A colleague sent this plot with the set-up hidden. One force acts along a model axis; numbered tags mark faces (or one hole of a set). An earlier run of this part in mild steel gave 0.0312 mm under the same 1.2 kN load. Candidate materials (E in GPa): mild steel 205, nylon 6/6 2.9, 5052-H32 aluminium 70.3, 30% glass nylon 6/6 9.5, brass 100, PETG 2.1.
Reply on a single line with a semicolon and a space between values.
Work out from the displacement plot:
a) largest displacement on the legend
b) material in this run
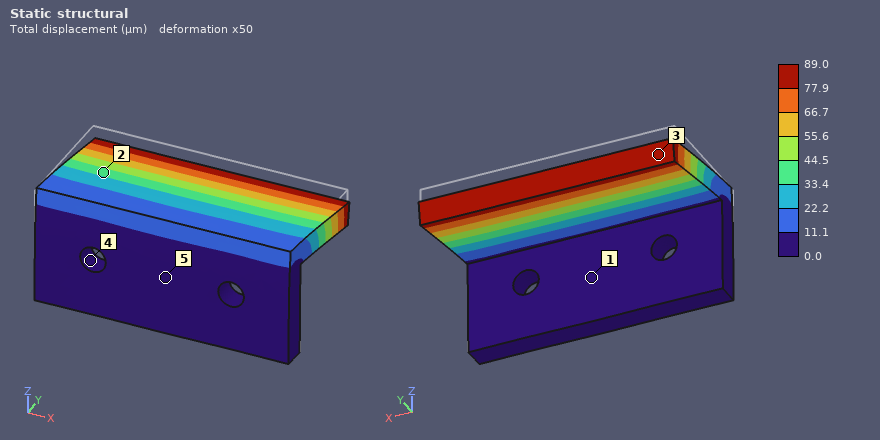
89.0 µm; 5052-H32 aluminium
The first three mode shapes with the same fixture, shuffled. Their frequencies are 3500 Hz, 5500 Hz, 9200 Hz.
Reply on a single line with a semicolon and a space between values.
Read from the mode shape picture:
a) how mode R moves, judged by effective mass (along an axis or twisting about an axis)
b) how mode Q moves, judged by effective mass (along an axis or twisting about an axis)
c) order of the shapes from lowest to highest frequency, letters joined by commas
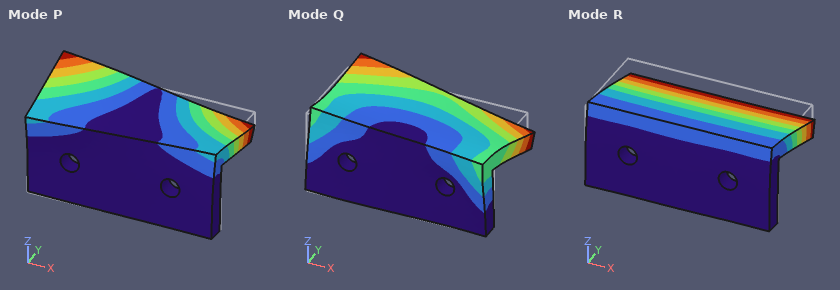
along Z; along X; R, P, Q
